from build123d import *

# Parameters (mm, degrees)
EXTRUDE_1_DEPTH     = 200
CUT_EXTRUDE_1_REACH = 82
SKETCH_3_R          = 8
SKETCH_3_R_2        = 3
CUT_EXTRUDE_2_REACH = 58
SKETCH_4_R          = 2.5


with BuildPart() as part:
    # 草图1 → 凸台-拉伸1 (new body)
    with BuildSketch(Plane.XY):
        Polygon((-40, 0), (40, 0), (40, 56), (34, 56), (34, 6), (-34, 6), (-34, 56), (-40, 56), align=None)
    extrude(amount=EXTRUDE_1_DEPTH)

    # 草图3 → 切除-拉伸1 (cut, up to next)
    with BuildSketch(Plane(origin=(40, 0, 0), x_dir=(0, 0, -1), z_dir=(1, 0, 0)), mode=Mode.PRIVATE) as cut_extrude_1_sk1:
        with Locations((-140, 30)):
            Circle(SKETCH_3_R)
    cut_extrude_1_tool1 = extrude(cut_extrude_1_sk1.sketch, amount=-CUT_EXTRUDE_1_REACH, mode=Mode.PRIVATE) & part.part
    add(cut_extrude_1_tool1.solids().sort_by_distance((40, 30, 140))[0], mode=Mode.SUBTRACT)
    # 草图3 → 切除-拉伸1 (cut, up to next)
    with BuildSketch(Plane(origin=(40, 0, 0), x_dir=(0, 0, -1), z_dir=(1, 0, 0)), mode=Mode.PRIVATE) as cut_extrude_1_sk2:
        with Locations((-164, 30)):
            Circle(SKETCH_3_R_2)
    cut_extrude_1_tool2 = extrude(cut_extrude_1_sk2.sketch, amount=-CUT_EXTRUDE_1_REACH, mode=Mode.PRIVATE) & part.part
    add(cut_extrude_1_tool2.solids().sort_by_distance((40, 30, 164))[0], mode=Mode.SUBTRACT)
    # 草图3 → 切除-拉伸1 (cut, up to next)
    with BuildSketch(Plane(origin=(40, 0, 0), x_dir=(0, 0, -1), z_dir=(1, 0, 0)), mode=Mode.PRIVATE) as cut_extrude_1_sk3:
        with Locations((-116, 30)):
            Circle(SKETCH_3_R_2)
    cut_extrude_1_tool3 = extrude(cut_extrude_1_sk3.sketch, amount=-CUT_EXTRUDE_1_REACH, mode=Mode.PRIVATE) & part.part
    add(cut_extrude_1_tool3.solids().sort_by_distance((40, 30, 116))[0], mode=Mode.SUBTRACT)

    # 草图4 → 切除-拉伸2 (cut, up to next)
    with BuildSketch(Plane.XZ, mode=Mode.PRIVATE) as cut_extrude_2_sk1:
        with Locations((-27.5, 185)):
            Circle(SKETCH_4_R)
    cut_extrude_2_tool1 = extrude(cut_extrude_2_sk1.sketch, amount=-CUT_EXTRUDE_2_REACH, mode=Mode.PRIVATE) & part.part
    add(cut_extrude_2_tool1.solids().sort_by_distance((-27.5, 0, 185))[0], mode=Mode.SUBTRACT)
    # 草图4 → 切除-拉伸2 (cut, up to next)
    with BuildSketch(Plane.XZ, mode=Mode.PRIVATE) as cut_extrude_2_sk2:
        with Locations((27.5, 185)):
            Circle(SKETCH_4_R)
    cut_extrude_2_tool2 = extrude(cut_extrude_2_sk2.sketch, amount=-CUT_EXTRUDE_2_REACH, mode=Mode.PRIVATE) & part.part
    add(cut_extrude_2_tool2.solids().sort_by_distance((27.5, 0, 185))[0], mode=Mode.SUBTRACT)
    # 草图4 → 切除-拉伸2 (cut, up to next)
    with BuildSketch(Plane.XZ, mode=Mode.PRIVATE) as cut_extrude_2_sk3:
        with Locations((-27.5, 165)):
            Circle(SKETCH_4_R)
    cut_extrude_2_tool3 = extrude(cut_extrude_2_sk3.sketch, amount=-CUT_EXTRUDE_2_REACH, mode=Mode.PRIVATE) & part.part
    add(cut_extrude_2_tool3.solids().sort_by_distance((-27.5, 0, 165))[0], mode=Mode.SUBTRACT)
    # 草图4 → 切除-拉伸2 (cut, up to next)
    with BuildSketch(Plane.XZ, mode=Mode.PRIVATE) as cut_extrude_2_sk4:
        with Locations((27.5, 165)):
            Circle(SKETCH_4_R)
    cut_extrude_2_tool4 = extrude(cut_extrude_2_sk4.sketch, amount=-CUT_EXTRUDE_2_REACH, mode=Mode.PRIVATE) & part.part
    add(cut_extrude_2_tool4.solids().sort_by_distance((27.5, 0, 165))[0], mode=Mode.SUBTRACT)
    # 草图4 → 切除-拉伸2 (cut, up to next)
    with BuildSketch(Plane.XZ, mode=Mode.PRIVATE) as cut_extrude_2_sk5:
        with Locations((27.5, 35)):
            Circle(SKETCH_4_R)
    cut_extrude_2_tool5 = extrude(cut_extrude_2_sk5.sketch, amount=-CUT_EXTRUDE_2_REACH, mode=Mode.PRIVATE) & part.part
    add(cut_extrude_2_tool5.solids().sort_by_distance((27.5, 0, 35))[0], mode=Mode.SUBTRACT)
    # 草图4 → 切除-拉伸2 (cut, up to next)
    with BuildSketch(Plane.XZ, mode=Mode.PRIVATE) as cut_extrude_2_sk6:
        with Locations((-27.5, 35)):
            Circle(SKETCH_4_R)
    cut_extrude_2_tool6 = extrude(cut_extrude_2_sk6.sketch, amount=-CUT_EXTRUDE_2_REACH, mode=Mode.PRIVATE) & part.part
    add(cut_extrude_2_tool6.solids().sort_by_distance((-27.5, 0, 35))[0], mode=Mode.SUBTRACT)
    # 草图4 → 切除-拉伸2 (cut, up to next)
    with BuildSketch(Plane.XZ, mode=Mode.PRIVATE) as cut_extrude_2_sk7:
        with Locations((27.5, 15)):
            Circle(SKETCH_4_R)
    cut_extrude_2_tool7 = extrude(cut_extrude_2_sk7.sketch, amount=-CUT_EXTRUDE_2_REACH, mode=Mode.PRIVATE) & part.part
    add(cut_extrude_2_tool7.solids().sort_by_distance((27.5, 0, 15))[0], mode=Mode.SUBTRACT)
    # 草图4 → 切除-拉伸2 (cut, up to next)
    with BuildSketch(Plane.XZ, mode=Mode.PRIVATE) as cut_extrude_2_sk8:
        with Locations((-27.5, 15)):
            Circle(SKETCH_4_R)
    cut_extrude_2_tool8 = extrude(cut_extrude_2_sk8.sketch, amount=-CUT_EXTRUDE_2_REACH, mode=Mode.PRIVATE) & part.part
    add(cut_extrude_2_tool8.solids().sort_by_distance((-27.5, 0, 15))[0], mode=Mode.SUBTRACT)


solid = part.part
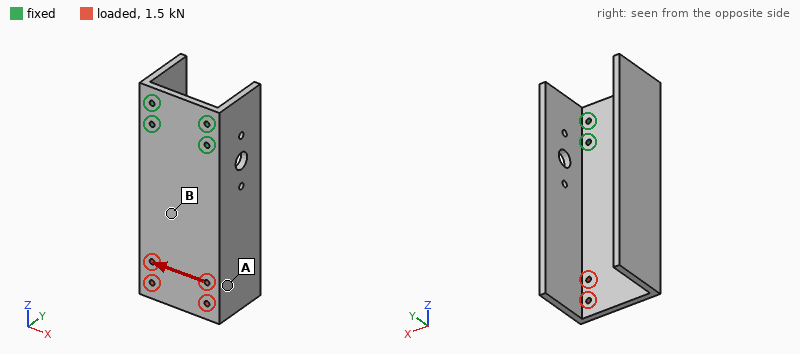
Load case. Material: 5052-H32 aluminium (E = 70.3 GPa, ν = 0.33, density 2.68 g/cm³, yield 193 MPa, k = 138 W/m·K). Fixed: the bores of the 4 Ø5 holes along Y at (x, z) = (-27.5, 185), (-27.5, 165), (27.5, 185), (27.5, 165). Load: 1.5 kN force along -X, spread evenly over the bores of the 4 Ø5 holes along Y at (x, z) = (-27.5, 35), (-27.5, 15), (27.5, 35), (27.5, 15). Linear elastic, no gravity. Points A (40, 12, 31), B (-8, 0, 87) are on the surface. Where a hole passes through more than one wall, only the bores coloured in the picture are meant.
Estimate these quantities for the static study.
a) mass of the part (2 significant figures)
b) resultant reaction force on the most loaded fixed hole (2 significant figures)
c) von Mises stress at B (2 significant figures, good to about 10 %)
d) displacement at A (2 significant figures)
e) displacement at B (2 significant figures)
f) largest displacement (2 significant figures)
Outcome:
570 g
2.7 kN
5.2 MPa
0.082 mm
0.033 mm
0.13 mm
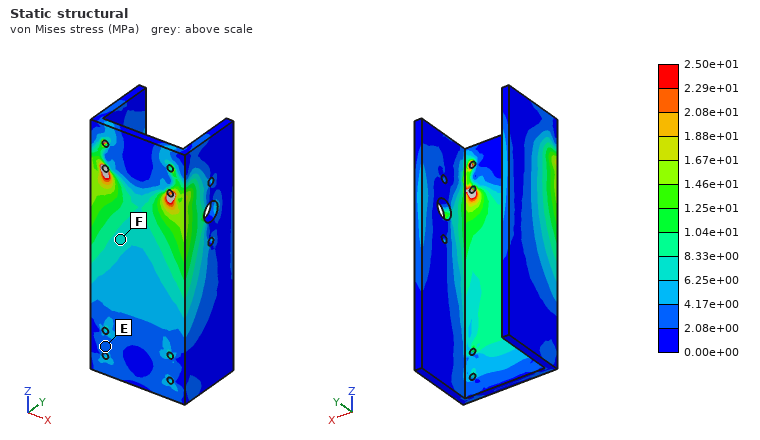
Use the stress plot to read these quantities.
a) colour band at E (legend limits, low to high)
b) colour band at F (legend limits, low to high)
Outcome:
2.08e+00 to 4.17e+00 MPa
6.25e+00 to 8.33e+00 MPa
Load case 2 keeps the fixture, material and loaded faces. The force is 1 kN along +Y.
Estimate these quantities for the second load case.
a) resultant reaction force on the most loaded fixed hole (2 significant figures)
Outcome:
3.1 kN
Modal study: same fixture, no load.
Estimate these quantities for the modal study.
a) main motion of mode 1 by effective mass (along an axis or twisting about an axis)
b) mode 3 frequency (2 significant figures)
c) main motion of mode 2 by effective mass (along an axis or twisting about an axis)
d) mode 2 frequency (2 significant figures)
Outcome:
along Y
1000 Hz
along X
580 Hz
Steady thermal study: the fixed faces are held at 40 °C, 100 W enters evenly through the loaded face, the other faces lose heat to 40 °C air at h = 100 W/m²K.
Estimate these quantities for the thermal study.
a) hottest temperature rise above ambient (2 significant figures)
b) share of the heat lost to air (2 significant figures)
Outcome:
42 K
89 %
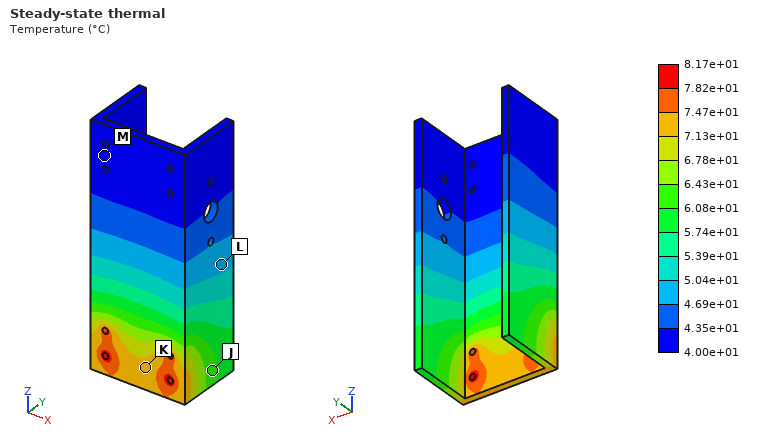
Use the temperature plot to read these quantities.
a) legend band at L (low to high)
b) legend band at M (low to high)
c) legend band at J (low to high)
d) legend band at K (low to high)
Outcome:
4.69e+01 to 5.04e+01 °C
4.00e+01 to 4.35e+01 °C
6.08e+01 to 6.43e+01 °C
7.13e+01 to 7.47e+01 °C
